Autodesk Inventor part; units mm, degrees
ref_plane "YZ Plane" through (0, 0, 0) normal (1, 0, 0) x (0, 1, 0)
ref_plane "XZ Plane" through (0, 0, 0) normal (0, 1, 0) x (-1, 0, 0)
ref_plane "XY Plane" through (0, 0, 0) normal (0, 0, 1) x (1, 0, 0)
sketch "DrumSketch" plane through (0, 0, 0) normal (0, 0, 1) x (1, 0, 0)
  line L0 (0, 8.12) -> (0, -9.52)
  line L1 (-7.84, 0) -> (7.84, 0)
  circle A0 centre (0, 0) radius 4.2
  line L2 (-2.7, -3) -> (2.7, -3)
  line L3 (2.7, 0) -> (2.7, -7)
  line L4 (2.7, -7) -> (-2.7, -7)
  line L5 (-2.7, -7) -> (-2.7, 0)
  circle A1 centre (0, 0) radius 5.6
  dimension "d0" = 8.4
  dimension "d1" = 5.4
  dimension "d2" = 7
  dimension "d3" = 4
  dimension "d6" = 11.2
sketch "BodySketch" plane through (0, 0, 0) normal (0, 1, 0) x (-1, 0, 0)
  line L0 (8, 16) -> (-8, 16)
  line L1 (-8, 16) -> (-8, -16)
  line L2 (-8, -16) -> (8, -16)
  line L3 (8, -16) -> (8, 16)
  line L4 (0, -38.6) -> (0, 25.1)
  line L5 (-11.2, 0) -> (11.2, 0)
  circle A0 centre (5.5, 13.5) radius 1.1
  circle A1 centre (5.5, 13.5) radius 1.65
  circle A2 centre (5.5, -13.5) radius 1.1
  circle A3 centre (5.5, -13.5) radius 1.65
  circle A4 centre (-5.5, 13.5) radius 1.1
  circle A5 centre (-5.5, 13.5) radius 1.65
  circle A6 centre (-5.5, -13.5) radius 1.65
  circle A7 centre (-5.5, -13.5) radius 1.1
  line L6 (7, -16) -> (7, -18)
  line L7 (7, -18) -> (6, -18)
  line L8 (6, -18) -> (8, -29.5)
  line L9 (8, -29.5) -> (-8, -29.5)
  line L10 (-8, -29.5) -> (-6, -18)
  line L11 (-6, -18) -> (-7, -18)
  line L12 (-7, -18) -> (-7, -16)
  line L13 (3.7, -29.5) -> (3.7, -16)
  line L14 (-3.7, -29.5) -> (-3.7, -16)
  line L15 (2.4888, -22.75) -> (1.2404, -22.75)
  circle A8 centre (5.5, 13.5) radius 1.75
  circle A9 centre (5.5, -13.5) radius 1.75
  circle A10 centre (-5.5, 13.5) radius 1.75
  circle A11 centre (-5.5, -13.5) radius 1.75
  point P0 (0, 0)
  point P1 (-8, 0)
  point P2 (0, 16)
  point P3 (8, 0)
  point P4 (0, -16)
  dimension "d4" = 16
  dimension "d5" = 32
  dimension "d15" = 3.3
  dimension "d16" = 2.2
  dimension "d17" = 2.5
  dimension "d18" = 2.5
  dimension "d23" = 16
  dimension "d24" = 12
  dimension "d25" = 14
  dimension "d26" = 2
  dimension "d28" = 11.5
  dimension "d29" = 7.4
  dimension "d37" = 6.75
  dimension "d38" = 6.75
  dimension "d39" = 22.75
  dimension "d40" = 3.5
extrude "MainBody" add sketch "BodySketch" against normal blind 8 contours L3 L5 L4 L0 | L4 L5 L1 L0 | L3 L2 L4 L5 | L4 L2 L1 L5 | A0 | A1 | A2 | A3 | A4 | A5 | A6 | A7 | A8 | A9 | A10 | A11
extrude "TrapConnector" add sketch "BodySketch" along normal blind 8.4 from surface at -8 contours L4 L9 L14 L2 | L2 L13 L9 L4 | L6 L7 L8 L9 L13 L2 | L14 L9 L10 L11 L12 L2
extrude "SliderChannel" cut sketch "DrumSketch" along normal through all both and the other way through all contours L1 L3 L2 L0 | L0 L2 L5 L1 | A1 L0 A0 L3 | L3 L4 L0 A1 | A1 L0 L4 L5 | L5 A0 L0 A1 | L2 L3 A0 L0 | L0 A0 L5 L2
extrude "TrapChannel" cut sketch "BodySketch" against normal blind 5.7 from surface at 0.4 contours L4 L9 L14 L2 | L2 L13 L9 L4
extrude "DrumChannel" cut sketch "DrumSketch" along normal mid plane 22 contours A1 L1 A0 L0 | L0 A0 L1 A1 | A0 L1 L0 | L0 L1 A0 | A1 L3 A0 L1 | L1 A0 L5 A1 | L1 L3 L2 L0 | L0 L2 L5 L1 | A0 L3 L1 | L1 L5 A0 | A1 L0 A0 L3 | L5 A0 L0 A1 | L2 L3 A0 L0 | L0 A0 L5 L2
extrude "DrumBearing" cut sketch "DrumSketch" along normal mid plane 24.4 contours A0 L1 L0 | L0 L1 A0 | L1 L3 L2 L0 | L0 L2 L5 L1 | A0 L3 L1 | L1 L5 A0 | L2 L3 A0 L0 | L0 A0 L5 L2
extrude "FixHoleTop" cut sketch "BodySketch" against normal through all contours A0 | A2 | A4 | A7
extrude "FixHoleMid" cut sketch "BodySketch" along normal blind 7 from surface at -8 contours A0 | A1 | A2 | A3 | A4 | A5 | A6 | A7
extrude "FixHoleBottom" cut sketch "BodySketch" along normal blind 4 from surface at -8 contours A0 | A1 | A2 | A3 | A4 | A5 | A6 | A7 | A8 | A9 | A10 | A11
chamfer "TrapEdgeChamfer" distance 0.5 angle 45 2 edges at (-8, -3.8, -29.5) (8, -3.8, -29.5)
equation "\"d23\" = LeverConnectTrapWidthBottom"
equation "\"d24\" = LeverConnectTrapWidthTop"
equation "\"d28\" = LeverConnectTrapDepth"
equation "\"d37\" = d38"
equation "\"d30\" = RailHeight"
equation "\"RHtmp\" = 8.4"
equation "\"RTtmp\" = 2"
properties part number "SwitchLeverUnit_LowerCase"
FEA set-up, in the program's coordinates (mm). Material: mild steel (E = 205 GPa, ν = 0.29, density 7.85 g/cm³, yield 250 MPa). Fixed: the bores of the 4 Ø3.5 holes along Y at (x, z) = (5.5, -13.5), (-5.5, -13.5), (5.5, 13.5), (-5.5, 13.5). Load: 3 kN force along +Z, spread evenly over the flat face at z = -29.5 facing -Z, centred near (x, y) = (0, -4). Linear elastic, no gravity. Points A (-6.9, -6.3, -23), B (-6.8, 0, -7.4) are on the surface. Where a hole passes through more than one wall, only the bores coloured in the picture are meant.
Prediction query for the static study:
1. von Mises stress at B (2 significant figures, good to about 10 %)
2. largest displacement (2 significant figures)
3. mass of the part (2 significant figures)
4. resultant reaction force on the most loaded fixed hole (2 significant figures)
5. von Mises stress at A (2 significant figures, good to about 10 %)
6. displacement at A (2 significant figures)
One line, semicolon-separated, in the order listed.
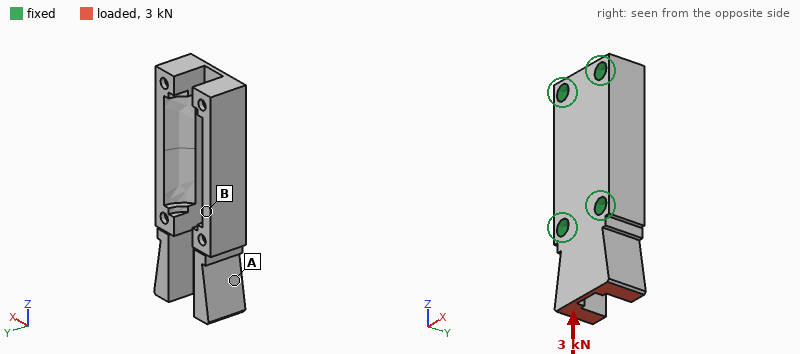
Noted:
15 MPa; 8.5 µm; 24 g; 1.4 kN; 54 MPa; 3.6 µm
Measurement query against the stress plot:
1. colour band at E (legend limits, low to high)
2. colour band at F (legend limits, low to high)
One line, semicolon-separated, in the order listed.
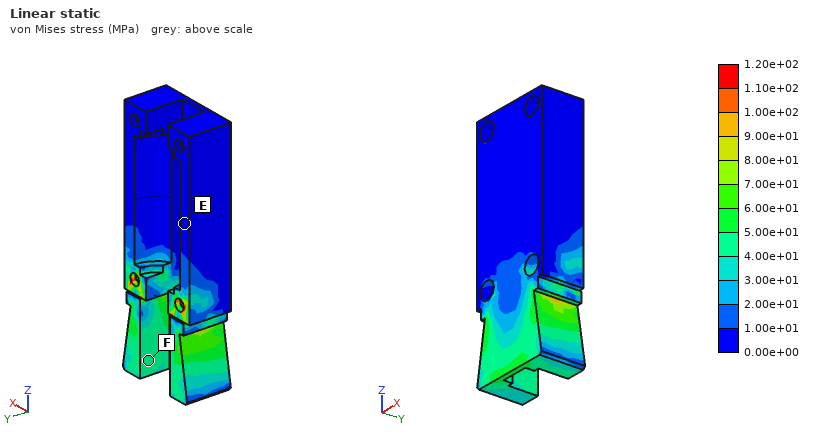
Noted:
0.00e+00 to 1.00e+01 MPa; 4.00e+01 to 5.00e+01 MPa
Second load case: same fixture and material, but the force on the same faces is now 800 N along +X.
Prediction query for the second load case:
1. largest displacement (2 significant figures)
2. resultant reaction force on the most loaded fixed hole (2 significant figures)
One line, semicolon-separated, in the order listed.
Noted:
33 µm; 950 N
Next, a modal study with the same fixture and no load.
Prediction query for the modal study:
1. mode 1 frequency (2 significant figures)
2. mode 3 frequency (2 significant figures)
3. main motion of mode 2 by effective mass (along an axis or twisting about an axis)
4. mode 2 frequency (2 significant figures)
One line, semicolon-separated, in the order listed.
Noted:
16 kHz; 21 kHz; along Y; 18 kHz
